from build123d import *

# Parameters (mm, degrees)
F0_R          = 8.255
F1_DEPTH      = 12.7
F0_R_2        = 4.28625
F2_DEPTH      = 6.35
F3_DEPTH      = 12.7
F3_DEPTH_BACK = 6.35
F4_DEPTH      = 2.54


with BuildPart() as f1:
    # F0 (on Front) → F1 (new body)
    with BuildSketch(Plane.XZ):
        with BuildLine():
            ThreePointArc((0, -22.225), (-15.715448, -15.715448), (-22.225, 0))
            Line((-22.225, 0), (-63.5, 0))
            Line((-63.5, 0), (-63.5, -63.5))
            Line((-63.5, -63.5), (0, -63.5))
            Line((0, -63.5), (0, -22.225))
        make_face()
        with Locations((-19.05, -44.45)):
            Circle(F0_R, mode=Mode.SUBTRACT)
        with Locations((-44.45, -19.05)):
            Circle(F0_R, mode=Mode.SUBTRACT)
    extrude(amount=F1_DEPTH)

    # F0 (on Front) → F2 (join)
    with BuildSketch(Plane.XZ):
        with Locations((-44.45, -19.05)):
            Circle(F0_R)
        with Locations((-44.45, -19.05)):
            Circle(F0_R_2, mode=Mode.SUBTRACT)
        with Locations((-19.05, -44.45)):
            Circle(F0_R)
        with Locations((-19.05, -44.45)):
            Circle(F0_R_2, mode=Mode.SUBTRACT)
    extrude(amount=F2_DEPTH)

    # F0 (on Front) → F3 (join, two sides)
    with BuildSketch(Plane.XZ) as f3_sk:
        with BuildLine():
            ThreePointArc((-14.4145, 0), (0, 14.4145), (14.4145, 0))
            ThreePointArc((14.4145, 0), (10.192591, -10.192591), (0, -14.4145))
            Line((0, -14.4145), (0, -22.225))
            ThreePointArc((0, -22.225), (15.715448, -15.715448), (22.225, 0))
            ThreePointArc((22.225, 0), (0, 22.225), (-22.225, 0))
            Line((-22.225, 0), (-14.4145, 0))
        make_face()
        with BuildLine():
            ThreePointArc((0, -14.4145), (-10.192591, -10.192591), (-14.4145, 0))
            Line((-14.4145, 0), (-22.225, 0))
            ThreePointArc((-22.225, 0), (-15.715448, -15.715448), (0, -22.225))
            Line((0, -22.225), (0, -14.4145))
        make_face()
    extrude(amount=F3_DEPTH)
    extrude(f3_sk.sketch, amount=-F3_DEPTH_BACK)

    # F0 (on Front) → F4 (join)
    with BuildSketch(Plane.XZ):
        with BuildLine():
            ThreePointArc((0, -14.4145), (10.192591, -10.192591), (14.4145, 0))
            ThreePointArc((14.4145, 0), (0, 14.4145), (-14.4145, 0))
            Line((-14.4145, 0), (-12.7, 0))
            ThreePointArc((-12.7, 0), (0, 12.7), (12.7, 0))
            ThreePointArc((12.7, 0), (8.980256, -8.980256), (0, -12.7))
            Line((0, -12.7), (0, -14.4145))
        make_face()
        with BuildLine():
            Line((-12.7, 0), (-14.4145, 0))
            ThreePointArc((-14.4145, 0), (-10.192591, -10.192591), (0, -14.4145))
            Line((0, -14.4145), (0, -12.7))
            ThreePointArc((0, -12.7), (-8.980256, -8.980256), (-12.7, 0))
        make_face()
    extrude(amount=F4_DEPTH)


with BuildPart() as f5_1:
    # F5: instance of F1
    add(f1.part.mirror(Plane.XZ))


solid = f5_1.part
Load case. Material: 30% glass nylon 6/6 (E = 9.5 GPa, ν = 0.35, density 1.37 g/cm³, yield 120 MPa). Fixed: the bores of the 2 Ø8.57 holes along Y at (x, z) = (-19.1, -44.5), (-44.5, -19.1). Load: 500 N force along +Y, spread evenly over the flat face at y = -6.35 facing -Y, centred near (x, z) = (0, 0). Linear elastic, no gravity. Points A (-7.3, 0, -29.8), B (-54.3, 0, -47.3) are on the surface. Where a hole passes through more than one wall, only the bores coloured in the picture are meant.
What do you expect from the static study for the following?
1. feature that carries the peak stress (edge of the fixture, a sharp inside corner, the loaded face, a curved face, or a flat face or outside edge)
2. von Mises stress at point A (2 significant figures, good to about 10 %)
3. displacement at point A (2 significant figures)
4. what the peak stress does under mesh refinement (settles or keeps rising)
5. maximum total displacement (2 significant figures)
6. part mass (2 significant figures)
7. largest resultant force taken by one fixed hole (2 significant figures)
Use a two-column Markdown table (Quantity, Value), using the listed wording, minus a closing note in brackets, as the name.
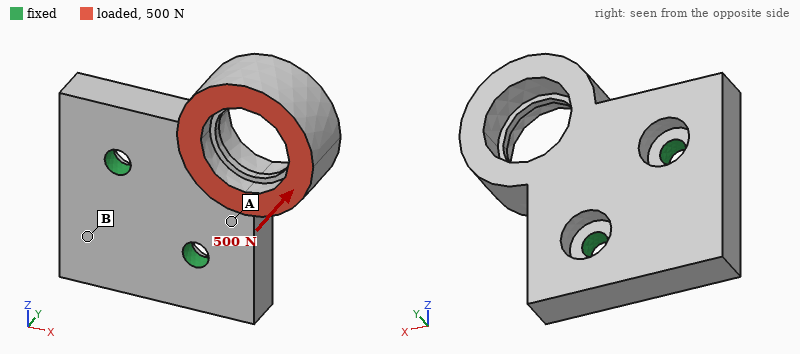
| Quantity | Value |
|---|---|
| feature that carries the peak stress | edge of the fixture |
| von Mises stress at point A | 10 MPa |
| displacement at point A | 0.10 mm |
| what the peak stress does under mesh refinement | keeps rising |
| maximum total displacement | 0.63 mm |
| part mass | 83 g |
| largest resultant force taken by one fixed hole | 310 N |
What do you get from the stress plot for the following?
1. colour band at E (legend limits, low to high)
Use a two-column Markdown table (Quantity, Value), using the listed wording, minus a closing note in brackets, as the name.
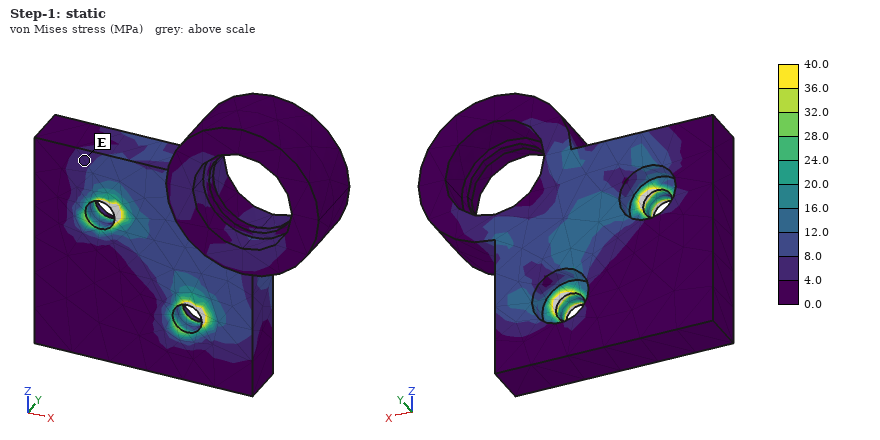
| Quantity | Value |
|---|---|
| colour band at E | 4.0 to 8.0 MPa |
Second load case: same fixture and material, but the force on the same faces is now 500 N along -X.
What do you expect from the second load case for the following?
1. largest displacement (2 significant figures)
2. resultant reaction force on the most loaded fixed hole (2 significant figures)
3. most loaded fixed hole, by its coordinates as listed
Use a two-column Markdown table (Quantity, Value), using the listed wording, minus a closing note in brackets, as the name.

| Quantity | Value |
|---|---|
| largest displacement | 0.19 mm |
| resultant reaction force on the most loaded fixed hole | 620 N |
| most loaded fixed hole, by its coordinates as listed | (-44.5, -19.1) |
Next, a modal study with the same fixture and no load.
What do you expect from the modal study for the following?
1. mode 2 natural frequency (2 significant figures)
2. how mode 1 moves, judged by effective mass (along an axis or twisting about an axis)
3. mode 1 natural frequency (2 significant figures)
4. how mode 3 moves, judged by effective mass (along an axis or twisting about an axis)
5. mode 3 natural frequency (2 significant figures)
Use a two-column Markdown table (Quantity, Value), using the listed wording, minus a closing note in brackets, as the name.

| Quantity | Value |
|---|---|
| mode 2 natural frequency | 2500 Hz |
| how mode 1 moves, judged by effective mass | along Y |
| mode 1 natural frequency | 1100 Hz |
| how mode 3 moves, judged by effective mass | along Y |
| mode 3 natural frequency | 3100 Hz |
